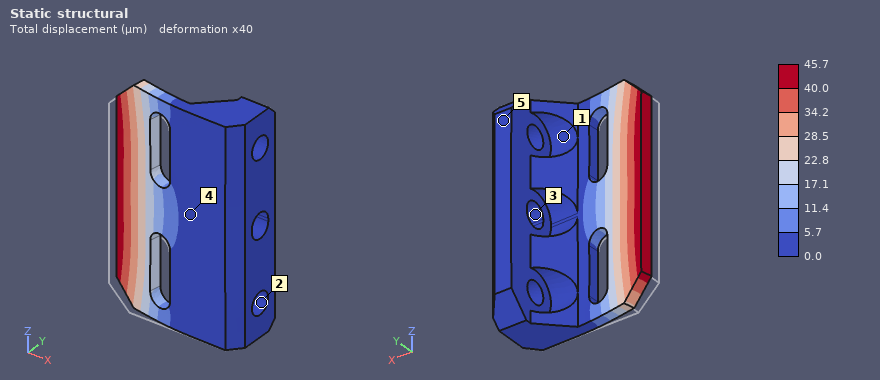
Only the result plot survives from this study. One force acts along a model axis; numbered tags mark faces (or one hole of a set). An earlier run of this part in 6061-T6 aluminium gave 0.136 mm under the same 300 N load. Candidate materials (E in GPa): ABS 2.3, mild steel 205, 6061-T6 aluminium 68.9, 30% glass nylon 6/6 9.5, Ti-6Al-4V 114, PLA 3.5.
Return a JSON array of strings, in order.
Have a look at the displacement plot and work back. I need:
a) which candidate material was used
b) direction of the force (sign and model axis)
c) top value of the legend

["mild steel", "+Y", "45.7 µm"]
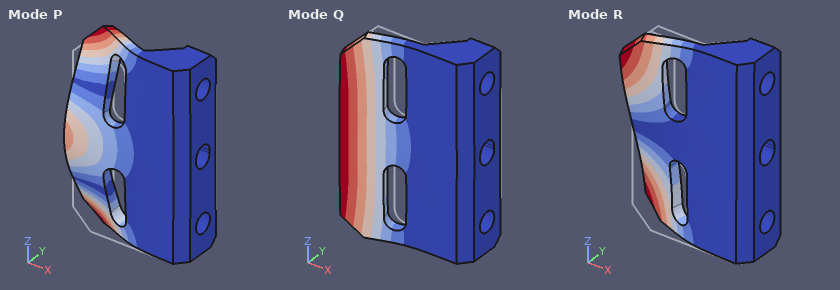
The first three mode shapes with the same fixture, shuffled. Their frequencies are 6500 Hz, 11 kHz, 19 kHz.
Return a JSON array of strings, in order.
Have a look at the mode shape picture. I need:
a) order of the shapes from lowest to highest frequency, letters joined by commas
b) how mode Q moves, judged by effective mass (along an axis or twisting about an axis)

["Q, R, P", "along Y"]
